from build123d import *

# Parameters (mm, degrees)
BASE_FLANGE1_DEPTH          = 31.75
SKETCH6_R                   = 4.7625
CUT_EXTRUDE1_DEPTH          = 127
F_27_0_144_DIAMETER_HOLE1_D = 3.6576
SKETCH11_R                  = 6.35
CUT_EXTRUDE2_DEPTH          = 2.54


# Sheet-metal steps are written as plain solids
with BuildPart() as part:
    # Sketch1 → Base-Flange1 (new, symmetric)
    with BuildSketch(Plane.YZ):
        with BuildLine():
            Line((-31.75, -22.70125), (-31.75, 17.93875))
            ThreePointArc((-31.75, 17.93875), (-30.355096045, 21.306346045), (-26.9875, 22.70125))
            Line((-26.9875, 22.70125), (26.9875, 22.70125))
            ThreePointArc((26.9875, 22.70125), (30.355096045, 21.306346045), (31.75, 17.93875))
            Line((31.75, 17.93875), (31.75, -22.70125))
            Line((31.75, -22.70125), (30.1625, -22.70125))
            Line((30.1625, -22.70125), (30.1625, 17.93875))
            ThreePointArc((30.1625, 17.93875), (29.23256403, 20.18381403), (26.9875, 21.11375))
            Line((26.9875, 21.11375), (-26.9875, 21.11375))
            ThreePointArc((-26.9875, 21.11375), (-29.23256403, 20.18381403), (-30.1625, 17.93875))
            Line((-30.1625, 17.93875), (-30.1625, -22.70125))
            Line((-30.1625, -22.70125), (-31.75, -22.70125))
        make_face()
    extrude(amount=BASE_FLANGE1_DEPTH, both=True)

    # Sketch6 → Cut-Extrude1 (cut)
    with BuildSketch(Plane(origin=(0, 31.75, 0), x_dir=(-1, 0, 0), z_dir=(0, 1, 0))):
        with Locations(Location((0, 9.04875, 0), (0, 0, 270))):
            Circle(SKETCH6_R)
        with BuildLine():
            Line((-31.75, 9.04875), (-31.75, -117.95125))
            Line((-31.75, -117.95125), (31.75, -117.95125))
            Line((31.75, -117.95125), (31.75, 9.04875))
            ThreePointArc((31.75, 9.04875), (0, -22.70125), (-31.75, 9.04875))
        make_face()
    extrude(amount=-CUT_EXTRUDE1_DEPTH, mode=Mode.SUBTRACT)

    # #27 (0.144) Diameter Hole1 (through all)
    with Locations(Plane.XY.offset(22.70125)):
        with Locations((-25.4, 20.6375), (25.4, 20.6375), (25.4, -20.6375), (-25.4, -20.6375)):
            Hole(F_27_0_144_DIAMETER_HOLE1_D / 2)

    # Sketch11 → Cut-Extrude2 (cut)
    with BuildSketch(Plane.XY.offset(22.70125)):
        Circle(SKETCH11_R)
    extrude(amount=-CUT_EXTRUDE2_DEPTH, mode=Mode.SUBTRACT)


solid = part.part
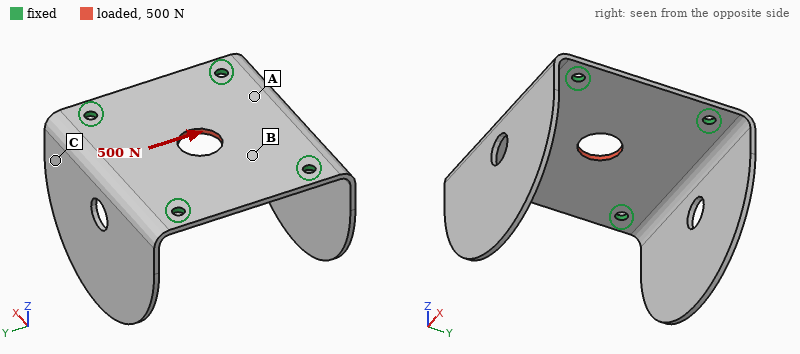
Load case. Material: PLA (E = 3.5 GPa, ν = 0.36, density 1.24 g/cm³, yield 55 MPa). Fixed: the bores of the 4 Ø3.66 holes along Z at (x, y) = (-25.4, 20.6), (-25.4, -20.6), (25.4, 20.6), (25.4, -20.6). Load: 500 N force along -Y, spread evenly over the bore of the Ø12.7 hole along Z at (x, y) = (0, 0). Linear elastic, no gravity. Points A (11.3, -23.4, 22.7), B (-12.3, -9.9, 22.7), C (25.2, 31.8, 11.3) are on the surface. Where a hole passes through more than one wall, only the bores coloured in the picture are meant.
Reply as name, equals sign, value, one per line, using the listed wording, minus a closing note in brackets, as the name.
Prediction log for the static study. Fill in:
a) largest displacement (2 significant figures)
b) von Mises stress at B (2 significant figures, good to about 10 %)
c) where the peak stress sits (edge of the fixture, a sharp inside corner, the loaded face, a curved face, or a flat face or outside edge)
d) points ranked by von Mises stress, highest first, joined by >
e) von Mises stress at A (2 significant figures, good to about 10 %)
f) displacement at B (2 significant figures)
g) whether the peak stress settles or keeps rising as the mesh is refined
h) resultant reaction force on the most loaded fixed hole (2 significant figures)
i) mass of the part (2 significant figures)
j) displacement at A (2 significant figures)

largest displacement = 70 µm
von Mises stress at B = 5.4 MPa
where the peak stress sits = edge of the fixture
points ranked by von Mises stress, highest first, joined by > = B > A > C
von Mises stress at A = 3.4 MPa
displacement at B = 38 µm
whether the peak stress settles or keeps rising as the mesh is refined = keeps rising
resultant reaction force on the most loaded fixed hole = 130 N
mass of the part = 16 g
displacement at A = 40 µm
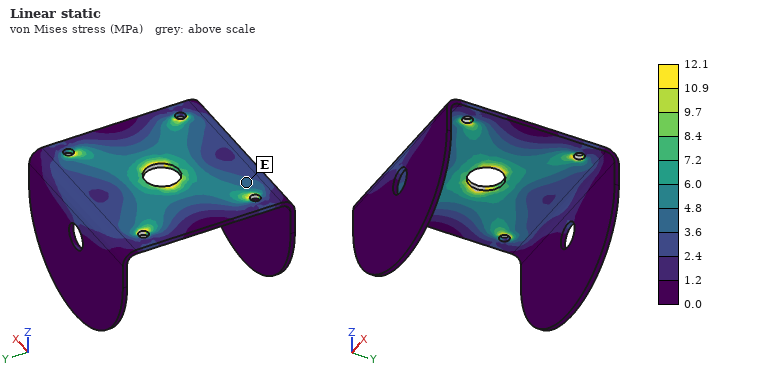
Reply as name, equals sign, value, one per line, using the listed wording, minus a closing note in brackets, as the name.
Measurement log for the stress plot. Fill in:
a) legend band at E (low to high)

legend band at E = 3.6 to 4.8 MPa
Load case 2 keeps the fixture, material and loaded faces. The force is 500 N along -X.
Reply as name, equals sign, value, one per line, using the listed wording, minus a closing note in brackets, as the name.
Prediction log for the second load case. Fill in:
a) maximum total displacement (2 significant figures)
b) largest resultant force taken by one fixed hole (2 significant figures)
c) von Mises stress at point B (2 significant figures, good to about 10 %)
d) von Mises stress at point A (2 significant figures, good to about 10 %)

maximum total displacement = 59 µm
largest resultant force taken by one fixed hole = 140 N
von Mises stress at point B = 5.7 MPa
von Mises stress at point A = 2.0 MPa
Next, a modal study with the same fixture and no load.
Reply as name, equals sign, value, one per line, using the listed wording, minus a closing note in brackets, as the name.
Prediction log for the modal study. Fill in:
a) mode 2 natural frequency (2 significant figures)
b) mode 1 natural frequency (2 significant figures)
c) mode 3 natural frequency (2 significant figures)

mode 2 natural frequency = 200 Hz
mode 1 natural frequency = 200 Hz
mode 3 natural frequency = 510 Hz
